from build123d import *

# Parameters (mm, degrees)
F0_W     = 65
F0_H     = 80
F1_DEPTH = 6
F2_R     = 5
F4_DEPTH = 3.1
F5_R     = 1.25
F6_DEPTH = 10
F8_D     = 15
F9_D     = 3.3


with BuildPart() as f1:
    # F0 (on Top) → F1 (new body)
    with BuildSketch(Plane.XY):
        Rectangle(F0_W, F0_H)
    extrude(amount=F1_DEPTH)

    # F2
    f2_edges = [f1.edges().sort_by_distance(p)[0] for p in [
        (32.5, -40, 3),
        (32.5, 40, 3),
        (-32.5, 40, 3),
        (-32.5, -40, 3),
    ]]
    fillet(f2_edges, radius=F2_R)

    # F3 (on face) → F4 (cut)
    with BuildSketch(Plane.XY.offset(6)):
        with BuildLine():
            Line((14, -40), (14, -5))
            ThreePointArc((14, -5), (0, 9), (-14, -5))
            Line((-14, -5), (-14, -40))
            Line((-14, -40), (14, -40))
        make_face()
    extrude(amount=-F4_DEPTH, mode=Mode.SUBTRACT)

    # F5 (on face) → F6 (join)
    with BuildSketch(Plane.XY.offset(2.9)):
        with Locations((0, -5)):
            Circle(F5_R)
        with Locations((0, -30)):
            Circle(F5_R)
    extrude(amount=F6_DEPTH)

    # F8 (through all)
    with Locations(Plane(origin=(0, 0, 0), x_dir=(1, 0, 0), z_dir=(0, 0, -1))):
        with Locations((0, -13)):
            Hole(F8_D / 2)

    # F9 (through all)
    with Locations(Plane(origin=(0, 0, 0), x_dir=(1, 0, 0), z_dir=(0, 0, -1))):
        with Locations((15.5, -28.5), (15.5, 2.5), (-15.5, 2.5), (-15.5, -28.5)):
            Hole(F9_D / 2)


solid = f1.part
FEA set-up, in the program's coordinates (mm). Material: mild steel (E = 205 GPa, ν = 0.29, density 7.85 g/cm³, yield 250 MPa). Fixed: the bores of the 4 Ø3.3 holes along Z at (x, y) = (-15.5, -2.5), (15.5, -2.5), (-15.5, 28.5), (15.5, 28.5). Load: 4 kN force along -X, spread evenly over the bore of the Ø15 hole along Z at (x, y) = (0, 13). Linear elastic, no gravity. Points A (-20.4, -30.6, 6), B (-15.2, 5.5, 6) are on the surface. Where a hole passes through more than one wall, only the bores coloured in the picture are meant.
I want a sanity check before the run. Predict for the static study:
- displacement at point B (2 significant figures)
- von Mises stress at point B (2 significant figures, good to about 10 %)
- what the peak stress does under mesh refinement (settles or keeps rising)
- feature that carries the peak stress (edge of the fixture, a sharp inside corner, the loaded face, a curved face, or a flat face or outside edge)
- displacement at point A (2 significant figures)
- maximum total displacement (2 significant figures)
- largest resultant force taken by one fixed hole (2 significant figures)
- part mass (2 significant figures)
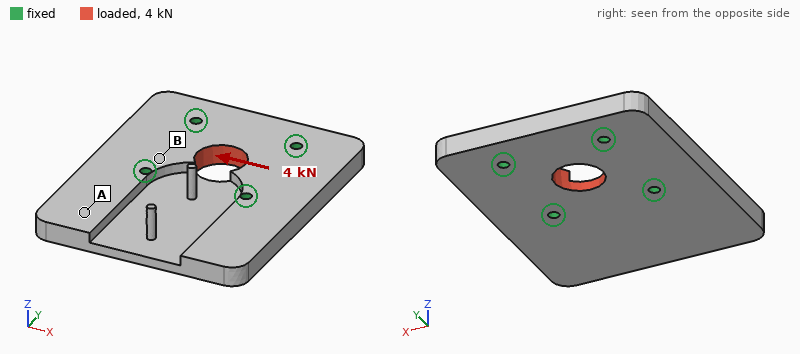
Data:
0.82 µm
8.8 MPa
keeps rising
edge of the fixture
0.26 µm
1.7 µm
1.2 kN
200 g
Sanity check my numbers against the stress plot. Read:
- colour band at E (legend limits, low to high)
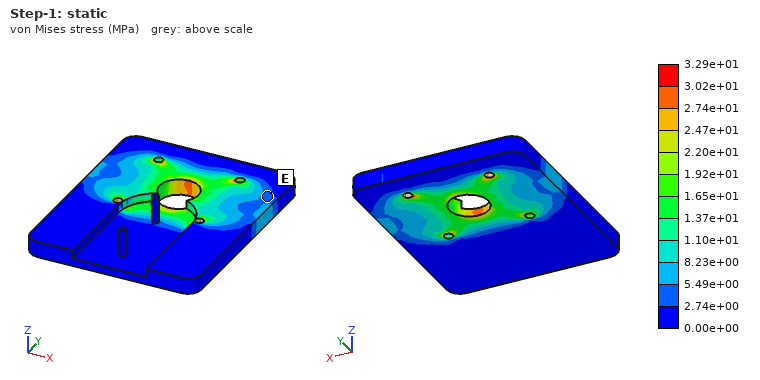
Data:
2.74e+00 to 5.49e+00 MPa
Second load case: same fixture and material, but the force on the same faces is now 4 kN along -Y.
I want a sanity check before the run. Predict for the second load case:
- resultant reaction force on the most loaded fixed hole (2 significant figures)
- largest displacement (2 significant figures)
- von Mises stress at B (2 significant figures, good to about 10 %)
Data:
1.2 kN
2.2 µm
9.9 MPa
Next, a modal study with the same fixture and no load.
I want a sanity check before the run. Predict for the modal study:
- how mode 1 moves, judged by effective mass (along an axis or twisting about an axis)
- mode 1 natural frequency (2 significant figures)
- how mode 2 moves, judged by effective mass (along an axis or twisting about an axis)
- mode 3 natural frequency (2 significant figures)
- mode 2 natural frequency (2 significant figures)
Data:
along Z
3000 Hz
twisting about Y
7200 Hz
3800 Hz
